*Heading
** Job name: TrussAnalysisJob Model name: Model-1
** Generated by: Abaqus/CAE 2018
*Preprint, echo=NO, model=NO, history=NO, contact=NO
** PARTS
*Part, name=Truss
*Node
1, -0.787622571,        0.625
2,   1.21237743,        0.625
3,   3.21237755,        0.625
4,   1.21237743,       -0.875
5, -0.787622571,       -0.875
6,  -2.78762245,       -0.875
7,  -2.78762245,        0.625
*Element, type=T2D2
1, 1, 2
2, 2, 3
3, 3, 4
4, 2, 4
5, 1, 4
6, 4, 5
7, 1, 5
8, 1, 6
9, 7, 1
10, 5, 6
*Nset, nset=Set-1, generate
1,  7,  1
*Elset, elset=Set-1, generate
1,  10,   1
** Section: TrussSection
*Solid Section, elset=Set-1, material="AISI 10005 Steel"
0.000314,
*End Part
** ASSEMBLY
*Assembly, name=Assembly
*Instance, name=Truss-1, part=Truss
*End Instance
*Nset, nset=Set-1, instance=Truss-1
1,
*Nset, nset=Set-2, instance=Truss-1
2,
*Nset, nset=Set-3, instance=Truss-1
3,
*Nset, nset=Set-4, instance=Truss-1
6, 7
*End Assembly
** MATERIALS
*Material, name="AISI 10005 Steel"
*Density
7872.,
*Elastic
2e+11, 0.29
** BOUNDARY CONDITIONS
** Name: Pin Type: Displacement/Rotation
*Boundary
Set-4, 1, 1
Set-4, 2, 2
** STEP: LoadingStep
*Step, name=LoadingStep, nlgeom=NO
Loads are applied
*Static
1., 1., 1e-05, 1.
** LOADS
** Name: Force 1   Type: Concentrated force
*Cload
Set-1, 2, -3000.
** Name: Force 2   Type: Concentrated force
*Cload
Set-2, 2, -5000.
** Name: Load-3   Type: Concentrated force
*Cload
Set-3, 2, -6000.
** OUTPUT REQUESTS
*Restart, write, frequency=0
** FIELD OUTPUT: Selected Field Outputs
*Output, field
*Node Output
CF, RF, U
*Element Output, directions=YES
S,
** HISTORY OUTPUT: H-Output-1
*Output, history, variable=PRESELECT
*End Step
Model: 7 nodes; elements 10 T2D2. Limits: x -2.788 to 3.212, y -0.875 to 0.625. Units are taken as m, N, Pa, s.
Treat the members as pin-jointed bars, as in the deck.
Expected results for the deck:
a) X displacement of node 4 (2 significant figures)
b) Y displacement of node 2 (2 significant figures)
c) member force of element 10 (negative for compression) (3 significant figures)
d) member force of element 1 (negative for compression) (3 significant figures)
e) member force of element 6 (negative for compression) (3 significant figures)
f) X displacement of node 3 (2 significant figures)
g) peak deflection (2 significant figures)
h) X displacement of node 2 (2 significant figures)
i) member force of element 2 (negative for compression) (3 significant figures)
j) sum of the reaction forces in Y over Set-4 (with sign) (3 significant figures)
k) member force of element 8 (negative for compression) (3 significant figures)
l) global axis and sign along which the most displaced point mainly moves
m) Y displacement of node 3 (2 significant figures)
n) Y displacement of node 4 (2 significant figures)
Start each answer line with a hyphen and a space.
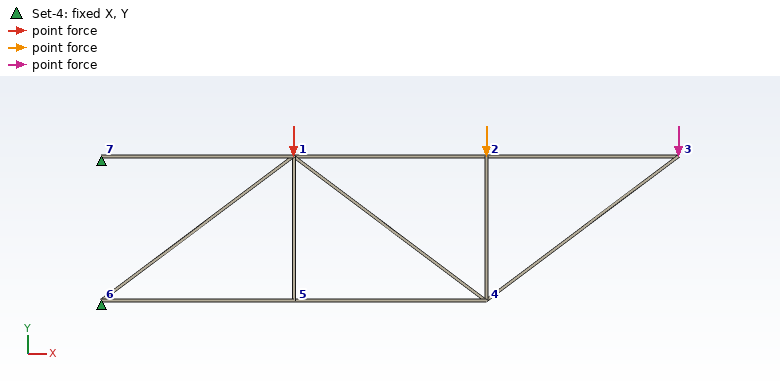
- -0.0014 m
- -0.0083 m
- -22700 N
- 8000 N
- -22700 N
- 0.0018 m
- 0.013 m
- 0.0016 m
- 8000 N
- 14000 N
- -23300 N
- -Y
- -0.013 m
- -0.0082 m
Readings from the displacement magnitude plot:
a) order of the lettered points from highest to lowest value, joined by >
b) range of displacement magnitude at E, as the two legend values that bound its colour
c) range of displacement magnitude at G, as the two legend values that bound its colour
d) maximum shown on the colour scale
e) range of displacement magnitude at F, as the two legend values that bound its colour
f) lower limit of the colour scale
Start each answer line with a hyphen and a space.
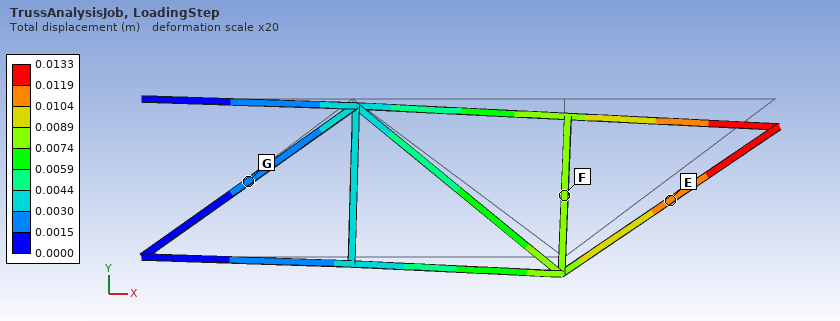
- E > F > G
- 0.0104 to 0.0119 m
- 0.0015 to 0.0030 m
- 0.0133 m
- 0.0074 to 0.0089 m
- 0.0000 m
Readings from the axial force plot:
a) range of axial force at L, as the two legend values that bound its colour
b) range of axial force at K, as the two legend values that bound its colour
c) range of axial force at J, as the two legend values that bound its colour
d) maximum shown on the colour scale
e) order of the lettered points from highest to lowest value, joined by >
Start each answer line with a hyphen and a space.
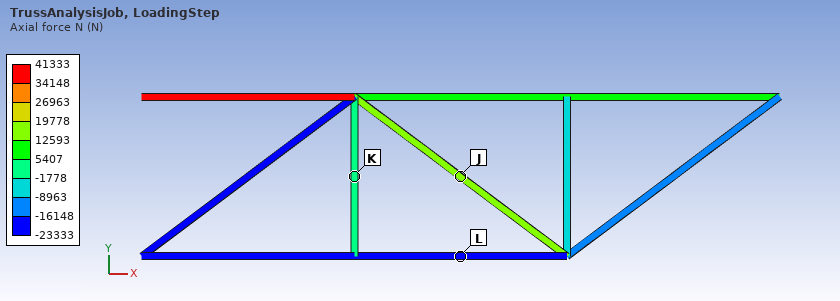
- -23333 to -16148 N
- -1778 to 5407 N
- 12593 to 19778 N
- 41333 N
- J > K > L
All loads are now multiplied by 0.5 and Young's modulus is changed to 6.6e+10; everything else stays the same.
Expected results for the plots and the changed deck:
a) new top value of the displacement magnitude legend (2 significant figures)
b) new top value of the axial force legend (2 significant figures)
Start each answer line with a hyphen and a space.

- 0.020 m
- 21000 N
